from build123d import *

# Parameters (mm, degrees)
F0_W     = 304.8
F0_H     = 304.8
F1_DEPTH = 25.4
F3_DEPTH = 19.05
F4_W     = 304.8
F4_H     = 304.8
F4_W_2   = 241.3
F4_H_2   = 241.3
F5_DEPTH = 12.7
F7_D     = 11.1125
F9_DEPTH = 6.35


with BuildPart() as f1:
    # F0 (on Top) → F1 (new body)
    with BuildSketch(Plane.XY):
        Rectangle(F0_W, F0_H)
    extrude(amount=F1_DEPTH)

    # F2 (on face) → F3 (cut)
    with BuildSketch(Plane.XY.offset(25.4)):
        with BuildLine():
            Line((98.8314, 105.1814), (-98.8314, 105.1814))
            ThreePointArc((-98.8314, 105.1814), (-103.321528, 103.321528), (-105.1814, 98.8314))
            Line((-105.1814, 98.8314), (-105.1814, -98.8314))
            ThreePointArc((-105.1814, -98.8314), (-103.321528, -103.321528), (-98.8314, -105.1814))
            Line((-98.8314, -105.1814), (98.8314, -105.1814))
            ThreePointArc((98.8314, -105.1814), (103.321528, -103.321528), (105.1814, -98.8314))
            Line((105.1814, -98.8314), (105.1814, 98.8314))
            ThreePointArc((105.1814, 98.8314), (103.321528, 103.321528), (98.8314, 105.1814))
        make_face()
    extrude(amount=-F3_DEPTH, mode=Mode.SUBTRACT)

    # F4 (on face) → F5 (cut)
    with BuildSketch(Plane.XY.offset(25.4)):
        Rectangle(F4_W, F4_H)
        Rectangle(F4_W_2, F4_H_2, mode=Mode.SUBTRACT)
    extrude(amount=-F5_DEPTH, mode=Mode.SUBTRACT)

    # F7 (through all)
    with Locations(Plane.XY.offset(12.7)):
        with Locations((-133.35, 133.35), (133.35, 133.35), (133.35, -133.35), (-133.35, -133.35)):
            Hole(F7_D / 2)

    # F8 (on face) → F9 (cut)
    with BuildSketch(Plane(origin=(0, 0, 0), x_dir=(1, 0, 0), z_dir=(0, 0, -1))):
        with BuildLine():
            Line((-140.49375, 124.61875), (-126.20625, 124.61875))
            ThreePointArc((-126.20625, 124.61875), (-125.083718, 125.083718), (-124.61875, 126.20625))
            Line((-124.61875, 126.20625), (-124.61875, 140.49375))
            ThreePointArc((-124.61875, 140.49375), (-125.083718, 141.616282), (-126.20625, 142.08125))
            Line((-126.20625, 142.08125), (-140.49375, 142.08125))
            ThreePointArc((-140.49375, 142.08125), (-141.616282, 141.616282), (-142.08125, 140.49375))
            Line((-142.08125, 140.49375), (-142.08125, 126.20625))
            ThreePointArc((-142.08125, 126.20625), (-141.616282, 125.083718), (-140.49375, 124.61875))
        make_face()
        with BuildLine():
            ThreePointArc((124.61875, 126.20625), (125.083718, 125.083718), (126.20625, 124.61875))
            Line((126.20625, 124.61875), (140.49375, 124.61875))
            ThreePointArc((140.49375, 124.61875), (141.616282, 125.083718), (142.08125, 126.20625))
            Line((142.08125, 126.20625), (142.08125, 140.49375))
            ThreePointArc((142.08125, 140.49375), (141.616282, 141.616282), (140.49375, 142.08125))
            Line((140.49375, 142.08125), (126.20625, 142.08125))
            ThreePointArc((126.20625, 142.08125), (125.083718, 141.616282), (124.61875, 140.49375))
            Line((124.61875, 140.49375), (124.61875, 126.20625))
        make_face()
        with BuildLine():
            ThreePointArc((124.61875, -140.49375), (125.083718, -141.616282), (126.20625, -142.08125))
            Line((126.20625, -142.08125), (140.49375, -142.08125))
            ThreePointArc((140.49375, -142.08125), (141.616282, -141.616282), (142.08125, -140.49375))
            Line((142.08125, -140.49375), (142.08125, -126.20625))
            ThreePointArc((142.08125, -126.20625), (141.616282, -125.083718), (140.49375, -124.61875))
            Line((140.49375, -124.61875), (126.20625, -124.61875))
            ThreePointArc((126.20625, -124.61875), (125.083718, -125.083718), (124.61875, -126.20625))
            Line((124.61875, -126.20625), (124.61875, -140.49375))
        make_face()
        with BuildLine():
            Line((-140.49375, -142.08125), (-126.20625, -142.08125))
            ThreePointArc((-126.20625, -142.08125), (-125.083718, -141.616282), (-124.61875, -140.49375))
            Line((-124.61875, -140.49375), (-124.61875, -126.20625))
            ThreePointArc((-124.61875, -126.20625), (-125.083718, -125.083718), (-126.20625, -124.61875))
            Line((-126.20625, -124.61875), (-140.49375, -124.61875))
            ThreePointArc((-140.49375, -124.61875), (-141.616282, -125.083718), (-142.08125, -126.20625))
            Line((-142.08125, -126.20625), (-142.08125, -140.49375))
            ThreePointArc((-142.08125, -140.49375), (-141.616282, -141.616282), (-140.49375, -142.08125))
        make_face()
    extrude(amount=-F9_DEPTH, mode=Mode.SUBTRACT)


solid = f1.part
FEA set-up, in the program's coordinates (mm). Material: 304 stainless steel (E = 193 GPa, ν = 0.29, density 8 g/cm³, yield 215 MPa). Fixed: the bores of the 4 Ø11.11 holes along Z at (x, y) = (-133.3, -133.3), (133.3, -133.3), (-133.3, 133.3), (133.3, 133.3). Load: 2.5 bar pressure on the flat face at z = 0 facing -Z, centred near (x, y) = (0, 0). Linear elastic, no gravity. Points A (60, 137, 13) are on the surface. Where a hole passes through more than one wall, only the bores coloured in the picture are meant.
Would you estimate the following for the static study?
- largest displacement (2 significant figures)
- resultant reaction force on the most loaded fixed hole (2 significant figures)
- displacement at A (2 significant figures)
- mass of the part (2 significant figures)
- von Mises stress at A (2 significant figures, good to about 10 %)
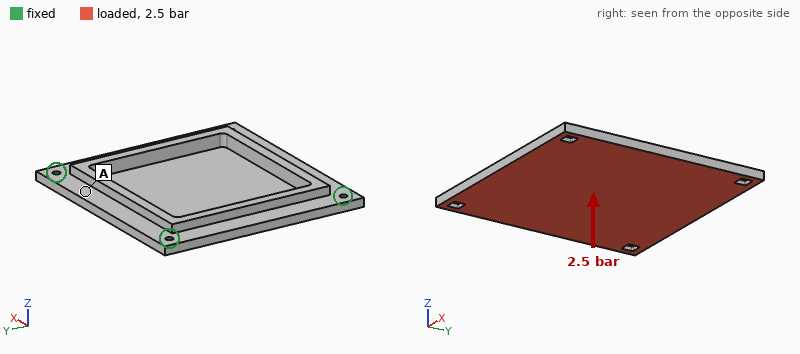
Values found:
0.47 mm
8.3 kN
0.11 mm
8.5 kg
17 MPa
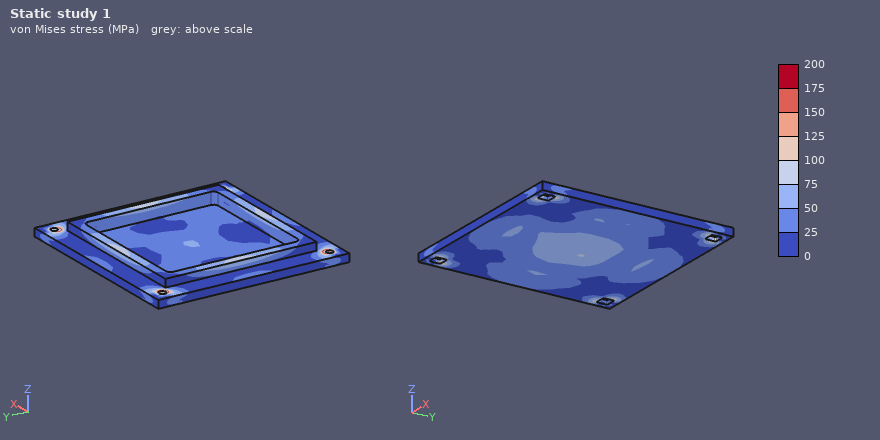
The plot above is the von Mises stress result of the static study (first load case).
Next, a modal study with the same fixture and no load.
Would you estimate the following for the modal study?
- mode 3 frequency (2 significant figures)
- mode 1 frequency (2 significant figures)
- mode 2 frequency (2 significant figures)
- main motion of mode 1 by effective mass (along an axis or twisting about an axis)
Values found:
960 Hz
600 Hz
950 Hz
along Z
